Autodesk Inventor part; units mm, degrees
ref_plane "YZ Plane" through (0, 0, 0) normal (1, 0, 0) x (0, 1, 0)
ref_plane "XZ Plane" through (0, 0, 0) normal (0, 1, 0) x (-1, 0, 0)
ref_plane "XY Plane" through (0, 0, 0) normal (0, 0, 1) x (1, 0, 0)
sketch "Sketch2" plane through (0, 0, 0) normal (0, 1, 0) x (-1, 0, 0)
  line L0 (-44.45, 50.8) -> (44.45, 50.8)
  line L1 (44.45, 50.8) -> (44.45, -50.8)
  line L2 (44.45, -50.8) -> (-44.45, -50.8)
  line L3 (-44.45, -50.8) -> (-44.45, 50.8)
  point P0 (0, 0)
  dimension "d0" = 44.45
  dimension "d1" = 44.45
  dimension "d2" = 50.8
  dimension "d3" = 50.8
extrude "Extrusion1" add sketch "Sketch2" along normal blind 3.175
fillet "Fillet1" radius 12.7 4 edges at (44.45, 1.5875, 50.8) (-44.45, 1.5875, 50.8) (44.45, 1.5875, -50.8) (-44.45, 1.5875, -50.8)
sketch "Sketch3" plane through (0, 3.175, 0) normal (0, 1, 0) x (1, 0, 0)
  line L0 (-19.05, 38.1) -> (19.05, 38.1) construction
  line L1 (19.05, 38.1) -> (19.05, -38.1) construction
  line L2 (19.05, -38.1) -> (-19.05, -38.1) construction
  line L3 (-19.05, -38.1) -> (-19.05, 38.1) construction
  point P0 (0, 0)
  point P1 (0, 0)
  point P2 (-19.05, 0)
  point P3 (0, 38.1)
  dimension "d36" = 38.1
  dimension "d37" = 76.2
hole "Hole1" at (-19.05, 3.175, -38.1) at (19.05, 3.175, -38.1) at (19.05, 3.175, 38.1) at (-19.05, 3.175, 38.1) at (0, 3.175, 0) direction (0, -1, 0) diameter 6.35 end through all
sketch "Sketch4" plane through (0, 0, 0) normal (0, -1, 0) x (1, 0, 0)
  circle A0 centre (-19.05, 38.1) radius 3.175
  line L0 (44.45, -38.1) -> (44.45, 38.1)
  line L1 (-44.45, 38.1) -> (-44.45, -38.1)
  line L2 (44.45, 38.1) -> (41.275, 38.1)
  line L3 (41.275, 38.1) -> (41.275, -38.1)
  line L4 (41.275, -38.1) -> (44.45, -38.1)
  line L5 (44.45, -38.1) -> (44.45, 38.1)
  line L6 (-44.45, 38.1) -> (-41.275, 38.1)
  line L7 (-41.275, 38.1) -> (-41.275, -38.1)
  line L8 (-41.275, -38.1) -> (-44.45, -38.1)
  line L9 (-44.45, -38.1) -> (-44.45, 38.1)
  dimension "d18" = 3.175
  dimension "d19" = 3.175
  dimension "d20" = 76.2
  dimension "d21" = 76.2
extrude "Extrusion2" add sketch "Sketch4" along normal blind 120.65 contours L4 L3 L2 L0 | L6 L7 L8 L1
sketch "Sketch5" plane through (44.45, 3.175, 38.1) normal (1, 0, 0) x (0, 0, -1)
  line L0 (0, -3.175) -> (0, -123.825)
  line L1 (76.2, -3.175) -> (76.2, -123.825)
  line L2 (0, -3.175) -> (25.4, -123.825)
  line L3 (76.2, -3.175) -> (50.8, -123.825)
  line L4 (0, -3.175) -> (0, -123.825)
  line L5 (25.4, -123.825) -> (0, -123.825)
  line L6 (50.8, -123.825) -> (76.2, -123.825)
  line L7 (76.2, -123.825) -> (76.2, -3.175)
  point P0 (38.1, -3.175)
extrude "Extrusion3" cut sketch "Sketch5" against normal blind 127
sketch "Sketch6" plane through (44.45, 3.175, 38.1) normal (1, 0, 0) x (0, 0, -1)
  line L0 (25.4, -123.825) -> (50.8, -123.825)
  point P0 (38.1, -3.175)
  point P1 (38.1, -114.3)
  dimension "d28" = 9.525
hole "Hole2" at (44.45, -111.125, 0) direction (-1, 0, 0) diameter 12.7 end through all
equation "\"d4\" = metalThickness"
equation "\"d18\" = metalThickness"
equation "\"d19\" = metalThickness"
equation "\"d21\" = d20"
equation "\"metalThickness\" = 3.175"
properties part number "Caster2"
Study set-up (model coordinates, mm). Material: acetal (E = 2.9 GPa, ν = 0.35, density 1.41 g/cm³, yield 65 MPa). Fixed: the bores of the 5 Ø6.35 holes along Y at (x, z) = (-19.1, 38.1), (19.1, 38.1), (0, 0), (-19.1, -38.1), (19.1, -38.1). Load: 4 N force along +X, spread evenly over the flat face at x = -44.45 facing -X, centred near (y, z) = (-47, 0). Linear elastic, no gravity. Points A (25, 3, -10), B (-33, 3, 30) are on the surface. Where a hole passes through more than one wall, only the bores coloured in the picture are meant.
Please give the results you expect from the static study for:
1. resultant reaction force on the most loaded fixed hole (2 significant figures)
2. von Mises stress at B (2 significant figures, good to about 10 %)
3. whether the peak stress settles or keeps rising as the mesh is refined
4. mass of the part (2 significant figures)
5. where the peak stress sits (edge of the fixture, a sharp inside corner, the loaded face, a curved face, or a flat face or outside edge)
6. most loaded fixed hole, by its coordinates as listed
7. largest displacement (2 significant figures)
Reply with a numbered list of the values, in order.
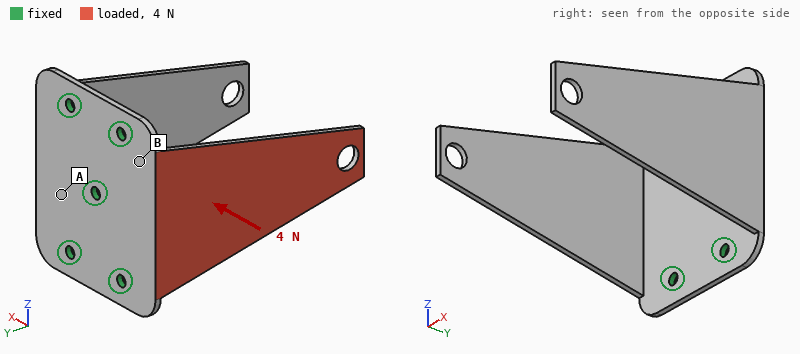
1. 4.0 N
2. 1.0 MPa
3. keeps rising
4. 93 g
5. edge of the fixture
6. (0, 0)
7. 1.9 mm
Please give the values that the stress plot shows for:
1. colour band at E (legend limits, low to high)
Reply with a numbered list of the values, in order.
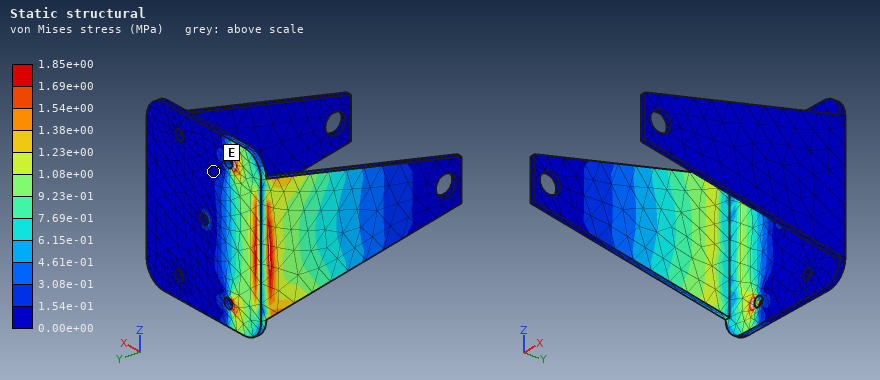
1. 0.00e+00 to 1.54e-01 MPa
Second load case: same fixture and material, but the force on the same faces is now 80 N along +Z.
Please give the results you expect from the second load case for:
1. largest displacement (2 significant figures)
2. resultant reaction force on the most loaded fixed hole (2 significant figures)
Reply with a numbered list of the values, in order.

1. 1.9 mm
2. 70 N
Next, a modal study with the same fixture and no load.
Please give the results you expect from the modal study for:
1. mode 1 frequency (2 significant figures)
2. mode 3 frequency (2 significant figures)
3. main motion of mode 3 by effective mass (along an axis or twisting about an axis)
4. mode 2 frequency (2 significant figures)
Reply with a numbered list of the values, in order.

1. 58 Hz
2. 230 Hz
3. along Z
4. 58 Hz
